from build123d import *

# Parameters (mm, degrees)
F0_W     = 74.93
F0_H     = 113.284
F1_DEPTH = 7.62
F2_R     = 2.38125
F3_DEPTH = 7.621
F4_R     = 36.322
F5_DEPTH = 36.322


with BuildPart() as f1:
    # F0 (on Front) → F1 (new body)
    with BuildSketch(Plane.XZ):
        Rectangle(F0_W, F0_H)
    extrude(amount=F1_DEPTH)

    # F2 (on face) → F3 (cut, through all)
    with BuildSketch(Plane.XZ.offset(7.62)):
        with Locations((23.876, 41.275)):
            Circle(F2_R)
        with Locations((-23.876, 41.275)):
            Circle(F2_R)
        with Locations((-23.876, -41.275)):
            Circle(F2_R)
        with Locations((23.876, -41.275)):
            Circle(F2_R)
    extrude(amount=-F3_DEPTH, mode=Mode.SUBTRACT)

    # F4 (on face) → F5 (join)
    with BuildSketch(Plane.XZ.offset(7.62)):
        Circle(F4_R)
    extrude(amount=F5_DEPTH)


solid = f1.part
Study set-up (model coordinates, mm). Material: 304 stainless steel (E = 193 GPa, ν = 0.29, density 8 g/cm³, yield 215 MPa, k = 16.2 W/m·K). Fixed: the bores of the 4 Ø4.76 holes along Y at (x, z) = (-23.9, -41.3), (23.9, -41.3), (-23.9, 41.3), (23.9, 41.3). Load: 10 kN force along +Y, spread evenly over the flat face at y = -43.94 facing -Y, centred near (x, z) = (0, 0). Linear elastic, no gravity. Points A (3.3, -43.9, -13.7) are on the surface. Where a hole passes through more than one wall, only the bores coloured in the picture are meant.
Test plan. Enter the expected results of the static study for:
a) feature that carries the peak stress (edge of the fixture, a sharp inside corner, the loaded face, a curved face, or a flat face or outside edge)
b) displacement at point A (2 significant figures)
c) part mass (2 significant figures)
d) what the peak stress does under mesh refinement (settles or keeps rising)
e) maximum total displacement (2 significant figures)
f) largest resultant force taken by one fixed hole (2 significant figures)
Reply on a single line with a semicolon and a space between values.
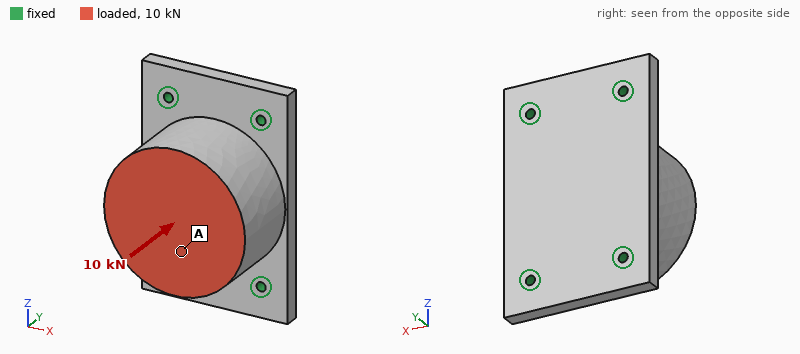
edge of the fixture; 8.7 µm; 1.7 kg; keeps rising; 9.0 µm; 2.7 kN
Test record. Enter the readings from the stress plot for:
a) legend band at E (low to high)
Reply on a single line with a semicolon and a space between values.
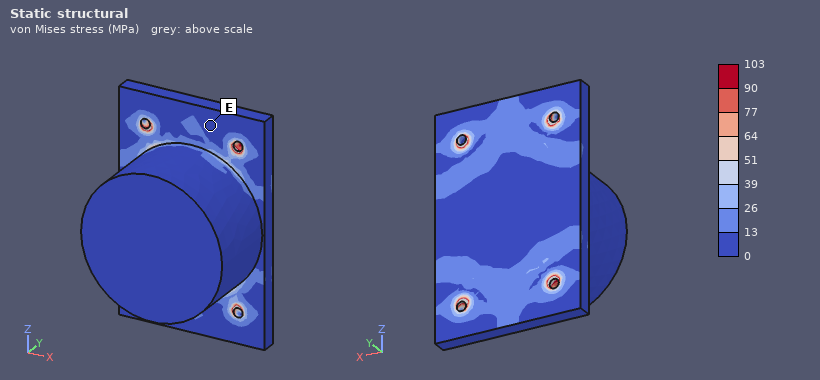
0 to 13 MPa
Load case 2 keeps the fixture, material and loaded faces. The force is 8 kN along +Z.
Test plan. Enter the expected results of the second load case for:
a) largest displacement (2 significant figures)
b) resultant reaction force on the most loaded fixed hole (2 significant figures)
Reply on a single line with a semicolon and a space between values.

12 µm; 3.0 kN
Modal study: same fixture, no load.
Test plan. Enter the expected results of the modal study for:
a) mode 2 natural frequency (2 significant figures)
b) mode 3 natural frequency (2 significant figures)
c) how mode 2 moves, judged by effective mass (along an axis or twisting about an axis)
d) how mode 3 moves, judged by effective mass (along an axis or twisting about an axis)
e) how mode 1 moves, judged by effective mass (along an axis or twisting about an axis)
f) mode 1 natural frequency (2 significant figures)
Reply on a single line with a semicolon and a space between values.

4500 Hz; 5600 Hz; along Y; along Z; along X; 3400 Hz
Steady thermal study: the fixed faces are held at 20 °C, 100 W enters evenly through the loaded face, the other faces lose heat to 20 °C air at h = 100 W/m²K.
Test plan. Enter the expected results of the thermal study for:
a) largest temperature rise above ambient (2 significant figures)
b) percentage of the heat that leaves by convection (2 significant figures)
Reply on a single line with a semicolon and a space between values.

84 K; 76 %
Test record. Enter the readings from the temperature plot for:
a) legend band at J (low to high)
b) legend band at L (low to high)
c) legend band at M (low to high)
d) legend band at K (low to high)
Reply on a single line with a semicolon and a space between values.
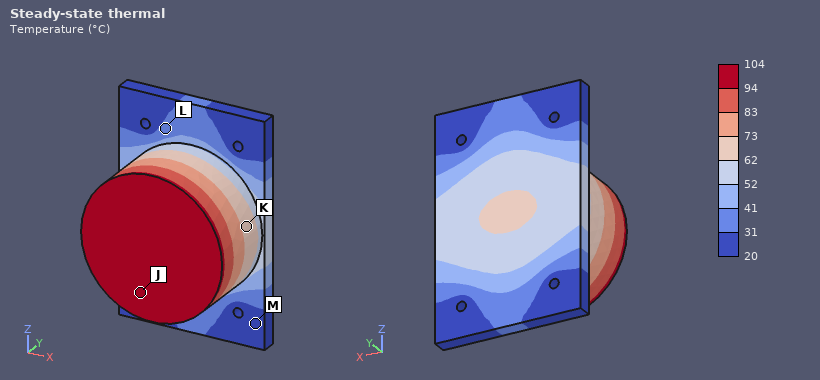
94 to 104 °C; 31 to 41 °C; 20 to 31 °C; 62 to 73 °C
